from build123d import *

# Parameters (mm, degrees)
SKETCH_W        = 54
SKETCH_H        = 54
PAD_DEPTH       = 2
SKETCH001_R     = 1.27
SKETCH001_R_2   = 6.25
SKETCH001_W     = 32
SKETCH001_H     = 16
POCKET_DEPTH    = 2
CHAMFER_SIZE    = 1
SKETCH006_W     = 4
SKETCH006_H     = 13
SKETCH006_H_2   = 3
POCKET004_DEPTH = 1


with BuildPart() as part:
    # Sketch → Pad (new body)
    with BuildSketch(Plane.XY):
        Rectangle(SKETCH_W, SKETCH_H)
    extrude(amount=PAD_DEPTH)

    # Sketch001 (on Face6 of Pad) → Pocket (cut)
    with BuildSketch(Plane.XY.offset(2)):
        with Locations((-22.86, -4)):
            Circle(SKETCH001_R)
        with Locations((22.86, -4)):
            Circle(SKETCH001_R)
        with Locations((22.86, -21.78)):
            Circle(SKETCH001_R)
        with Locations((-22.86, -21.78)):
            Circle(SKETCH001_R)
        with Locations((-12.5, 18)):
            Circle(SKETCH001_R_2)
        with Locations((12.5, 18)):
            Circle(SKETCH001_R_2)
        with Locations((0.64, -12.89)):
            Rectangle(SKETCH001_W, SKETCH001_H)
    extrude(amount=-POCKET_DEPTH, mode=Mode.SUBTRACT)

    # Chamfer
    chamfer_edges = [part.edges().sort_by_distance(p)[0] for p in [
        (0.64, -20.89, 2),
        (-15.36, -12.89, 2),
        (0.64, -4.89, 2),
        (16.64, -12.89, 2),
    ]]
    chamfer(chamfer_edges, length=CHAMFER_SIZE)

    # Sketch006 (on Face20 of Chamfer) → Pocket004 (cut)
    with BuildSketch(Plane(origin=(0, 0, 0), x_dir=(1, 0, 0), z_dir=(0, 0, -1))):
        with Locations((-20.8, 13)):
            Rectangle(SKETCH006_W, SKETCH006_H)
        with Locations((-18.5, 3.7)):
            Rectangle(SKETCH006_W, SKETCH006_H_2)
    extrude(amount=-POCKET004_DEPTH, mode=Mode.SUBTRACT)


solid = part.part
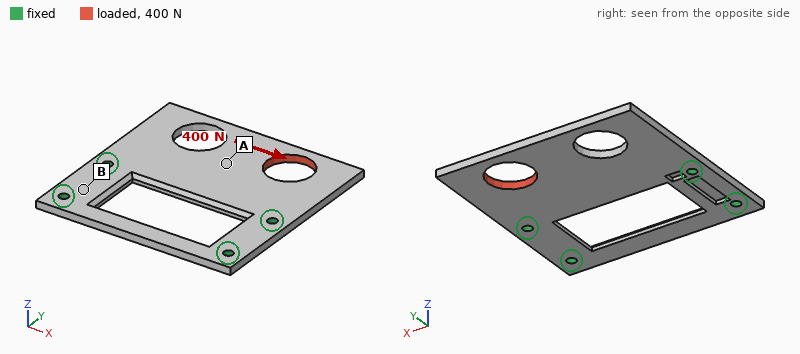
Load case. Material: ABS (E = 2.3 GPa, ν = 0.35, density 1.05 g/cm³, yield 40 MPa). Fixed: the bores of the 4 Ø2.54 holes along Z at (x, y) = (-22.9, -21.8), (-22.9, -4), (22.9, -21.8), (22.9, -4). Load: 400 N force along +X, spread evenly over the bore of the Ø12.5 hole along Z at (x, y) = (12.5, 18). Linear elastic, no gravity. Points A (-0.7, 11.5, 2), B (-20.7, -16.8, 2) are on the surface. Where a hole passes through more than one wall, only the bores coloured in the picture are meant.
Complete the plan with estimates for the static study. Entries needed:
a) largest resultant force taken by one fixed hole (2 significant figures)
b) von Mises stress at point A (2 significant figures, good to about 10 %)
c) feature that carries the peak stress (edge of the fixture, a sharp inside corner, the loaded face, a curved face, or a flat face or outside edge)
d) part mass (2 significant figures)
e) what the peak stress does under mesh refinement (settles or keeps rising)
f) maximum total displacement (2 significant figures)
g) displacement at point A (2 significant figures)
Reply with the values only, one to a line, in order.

270 N
7.6 MPa
edge of the fixture
4.4 g
keeps rising
0.40 mm
0.14 mm
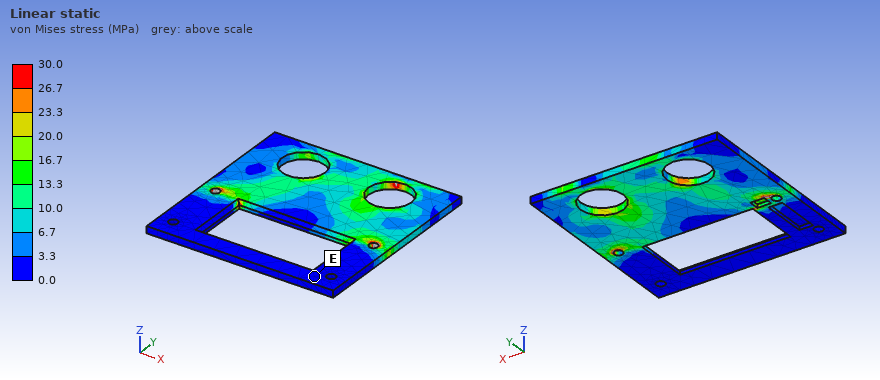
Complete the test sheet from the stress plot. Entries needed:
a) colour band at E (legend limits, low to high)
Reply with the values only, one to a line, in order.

0.0 to 3.3 MPa
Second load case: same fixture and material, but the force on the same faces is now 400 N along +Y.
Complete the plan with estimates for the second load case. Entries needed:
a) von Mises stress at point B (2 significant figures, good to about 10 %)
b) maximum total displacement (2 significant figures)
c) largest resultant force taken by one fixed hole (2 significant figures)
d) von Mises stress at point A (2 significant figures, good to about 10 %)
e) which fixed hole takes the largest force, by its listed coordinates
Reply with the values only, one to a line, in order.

2.7 MPa
0.23 mm
280 N
5.4 MPa
(22.9, -4)
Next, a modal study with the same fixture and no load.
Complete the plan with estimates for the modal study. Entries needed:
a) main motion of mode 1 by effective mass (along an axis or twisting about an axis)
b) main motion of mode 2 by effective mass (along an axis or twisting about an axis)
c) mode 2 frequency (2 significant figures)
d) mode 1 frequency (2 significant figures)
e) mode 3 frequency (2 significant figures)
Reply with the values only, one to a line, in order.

along Z
twisting about Y
810 Hz
400 Hz
1200 Hz
